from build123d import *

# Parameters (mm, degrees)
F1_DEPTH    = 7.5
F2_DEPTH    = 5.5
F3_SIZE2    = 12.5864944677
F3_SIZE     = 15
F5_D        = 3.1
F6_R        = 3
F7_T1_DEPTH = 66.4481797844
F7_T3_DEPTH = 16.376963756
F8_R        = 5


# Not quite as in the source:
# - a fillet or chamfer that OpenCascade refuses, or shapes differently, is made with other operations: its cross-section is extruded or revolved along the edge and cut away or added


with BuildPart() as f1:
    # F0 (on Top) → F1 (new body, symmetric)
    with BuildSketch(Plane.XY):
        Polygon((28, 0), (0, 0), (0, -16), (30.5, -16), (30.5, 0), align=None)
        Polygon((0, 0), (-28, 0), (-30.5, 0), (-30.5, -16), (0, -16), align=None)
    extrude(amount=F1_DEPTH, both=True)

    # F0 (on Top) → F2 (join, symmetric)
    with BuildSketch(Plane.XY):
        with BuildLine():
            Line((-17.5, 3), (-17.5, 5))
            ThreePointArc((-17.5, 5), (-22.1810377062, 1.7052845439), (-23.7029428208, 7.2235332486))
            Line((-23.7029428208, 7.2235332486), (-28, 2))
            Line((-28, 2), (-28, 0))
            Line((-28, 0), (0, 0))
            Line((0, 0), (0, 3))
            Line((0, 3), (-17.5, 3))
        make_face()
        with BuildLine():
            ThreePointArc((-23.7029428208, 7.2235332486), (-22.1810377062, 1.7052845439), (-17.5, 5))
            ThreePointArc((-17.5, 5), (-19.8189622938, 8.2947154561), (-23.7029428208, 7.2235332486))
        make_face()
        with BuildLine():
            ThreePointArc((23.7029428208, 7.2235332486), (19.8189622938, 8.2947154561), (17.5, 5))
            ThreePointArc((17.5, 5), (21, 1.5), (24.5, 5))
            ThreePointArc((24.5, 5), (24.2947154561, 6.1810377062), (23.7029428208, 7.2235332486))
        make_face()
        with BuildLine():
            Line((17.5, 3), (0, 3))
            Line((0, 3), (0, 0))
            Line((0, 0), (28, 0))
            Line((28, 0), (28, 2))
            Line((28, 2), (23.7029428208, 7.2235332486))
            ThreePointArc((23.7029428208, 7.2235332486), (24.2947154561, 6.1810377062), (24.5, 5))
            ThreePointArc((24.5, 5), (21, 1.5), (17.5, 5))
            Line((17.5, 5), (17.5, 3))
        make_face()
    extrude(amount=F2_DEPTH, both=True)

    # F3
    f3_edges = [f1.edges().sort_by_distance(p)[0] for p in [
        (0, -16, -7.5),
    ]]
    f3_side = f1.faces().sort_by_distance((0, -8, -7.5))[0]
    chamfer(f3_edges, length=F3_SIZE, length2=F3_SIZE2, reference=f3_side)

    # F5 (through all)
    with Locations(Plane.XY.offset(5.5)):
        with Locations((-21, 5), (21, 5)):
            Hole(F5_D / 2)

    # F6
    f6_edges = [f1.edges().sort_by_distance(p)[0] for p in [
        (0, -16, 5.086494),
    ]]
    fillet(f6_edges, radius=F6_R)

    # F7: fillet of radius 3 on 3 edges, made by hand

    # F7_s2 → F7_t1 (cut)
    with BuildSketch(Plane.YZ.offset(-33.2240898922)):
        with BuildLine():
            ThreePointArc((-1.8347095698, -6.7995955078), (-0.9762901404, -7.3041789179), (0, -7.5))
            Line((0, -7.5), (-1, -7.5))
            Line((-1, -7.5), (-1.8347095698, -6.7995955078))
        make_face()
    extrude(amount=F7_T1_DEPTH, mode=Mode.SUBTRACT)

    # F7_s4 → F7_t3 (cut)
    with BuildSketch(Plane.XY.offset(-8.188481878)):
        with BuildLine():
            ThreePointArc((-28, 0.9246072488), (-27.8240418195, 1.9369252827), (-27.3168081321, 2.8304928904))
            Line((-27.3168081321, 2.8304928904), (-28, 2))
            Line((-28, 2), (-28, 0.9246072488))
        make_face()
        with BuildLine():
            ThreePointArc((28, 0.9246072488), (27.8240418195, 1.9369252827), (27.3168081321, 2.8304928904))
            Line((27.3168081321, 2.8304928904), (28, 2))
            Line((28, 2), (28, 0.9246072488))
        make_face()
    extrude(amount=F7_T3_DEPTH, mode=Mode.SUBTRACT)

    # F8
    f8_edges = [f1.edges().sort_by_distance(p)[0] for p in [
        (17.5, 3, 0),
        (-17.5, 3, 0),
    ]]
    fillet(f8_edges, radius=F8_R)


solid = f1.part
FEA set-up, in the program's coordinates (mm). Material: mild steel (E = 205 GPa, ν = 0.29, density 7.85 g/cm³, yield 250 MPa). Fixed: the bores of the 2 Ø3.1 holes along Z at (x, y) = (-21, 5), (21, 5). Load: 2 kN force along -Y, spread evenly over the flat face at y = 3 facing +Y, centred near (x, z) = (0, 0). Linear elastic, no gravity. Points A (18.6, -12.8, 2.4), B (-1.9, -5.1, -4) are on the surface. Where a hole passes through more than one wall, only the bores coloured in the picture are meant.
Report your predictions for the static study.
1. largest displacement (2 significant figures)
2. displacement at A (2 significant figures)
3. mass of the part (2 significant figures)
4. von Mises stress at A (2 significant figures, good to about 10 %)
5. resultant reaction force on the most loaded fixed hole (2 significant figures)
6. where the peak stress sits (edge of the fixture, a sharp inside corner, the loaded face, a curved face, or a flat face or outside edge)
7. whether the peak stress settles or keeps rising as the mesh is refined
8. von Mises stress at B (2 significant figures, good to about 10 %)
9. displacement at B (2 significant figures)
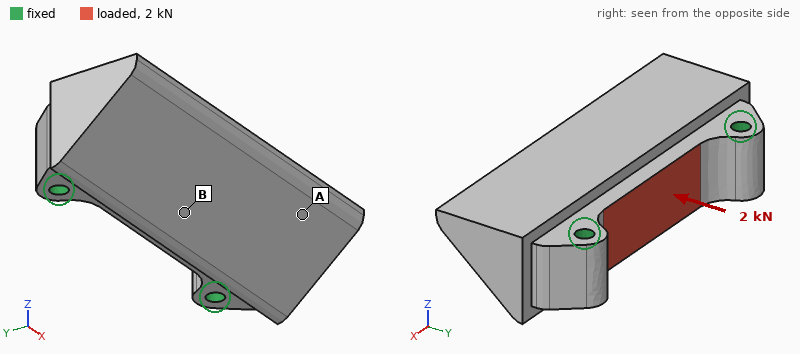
3.4 µm
1.1 µm
90 g
3.8 MPa
1.2 kN
edge of the fixture
keeps rising
17 MPa
2.9 µm
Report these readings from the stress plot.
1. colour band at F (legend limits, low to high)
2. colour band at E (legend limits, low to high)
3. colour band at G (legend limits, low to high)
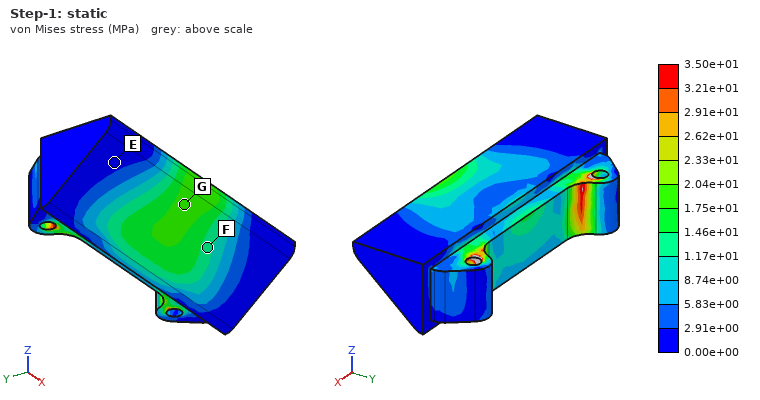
1.17e+01 to 1.46e+01 MPa
0.00e+00 to 2.91e+00 MPa
1.75e+01 to 2.04e+01 MPa
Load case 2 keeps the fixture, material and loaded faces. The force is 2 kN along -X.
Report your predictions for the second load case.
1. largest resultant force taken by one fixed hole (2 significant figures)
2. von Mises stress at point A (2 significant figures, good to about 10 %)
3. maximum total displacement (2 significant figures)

1.0 kN
5.7 MPa
1.8 µm
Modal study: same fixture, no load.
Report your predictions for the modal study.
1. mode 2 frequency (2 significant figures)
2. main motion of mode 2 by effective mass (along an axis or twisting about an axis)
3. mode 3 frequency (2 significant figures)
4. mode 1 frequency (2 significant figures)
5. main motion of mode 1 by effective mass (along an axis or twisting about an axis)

19 kHz
twisting about Y
21 kHz
12 kHz
along Z
